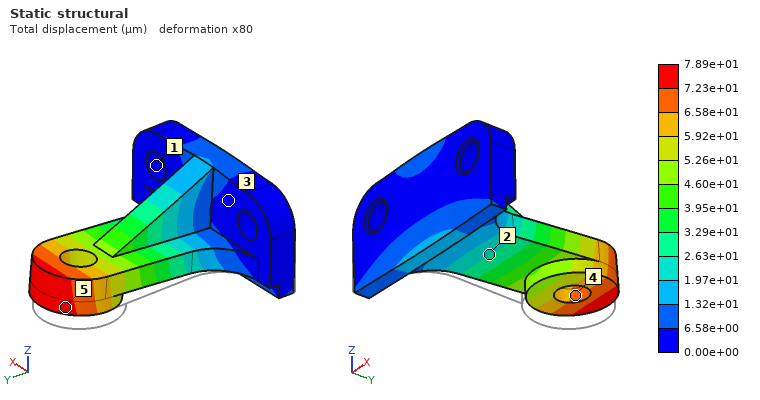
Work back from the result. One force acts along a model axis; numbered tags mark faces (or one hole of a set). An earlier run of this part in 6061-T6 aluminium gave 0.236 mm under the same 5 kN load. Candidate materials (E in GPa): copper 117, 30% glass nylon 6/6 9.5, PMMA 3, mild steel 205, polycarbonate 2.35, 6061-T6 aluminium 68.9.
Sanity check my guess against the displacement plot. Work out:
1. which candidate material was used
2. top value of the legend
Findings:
mild steel
7.89e+01 µm
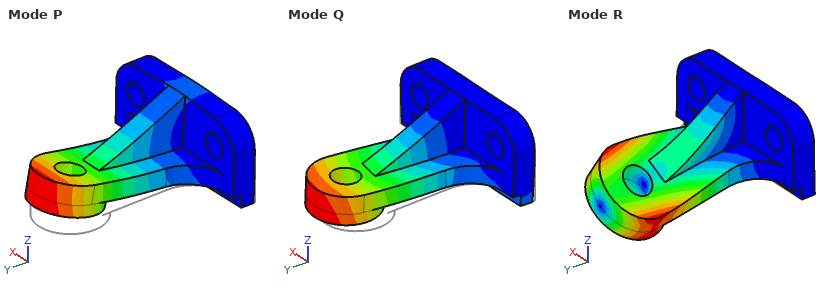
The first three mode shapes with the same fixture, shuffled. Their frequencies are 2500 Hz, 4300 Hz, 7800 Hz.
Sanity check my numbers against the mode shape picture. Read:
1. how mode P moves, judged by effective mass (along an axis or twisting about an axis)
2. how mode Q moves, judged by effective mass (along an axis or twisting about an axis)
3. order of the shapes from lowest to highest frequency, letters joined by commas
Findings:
along Z
along X
P, Q, R
